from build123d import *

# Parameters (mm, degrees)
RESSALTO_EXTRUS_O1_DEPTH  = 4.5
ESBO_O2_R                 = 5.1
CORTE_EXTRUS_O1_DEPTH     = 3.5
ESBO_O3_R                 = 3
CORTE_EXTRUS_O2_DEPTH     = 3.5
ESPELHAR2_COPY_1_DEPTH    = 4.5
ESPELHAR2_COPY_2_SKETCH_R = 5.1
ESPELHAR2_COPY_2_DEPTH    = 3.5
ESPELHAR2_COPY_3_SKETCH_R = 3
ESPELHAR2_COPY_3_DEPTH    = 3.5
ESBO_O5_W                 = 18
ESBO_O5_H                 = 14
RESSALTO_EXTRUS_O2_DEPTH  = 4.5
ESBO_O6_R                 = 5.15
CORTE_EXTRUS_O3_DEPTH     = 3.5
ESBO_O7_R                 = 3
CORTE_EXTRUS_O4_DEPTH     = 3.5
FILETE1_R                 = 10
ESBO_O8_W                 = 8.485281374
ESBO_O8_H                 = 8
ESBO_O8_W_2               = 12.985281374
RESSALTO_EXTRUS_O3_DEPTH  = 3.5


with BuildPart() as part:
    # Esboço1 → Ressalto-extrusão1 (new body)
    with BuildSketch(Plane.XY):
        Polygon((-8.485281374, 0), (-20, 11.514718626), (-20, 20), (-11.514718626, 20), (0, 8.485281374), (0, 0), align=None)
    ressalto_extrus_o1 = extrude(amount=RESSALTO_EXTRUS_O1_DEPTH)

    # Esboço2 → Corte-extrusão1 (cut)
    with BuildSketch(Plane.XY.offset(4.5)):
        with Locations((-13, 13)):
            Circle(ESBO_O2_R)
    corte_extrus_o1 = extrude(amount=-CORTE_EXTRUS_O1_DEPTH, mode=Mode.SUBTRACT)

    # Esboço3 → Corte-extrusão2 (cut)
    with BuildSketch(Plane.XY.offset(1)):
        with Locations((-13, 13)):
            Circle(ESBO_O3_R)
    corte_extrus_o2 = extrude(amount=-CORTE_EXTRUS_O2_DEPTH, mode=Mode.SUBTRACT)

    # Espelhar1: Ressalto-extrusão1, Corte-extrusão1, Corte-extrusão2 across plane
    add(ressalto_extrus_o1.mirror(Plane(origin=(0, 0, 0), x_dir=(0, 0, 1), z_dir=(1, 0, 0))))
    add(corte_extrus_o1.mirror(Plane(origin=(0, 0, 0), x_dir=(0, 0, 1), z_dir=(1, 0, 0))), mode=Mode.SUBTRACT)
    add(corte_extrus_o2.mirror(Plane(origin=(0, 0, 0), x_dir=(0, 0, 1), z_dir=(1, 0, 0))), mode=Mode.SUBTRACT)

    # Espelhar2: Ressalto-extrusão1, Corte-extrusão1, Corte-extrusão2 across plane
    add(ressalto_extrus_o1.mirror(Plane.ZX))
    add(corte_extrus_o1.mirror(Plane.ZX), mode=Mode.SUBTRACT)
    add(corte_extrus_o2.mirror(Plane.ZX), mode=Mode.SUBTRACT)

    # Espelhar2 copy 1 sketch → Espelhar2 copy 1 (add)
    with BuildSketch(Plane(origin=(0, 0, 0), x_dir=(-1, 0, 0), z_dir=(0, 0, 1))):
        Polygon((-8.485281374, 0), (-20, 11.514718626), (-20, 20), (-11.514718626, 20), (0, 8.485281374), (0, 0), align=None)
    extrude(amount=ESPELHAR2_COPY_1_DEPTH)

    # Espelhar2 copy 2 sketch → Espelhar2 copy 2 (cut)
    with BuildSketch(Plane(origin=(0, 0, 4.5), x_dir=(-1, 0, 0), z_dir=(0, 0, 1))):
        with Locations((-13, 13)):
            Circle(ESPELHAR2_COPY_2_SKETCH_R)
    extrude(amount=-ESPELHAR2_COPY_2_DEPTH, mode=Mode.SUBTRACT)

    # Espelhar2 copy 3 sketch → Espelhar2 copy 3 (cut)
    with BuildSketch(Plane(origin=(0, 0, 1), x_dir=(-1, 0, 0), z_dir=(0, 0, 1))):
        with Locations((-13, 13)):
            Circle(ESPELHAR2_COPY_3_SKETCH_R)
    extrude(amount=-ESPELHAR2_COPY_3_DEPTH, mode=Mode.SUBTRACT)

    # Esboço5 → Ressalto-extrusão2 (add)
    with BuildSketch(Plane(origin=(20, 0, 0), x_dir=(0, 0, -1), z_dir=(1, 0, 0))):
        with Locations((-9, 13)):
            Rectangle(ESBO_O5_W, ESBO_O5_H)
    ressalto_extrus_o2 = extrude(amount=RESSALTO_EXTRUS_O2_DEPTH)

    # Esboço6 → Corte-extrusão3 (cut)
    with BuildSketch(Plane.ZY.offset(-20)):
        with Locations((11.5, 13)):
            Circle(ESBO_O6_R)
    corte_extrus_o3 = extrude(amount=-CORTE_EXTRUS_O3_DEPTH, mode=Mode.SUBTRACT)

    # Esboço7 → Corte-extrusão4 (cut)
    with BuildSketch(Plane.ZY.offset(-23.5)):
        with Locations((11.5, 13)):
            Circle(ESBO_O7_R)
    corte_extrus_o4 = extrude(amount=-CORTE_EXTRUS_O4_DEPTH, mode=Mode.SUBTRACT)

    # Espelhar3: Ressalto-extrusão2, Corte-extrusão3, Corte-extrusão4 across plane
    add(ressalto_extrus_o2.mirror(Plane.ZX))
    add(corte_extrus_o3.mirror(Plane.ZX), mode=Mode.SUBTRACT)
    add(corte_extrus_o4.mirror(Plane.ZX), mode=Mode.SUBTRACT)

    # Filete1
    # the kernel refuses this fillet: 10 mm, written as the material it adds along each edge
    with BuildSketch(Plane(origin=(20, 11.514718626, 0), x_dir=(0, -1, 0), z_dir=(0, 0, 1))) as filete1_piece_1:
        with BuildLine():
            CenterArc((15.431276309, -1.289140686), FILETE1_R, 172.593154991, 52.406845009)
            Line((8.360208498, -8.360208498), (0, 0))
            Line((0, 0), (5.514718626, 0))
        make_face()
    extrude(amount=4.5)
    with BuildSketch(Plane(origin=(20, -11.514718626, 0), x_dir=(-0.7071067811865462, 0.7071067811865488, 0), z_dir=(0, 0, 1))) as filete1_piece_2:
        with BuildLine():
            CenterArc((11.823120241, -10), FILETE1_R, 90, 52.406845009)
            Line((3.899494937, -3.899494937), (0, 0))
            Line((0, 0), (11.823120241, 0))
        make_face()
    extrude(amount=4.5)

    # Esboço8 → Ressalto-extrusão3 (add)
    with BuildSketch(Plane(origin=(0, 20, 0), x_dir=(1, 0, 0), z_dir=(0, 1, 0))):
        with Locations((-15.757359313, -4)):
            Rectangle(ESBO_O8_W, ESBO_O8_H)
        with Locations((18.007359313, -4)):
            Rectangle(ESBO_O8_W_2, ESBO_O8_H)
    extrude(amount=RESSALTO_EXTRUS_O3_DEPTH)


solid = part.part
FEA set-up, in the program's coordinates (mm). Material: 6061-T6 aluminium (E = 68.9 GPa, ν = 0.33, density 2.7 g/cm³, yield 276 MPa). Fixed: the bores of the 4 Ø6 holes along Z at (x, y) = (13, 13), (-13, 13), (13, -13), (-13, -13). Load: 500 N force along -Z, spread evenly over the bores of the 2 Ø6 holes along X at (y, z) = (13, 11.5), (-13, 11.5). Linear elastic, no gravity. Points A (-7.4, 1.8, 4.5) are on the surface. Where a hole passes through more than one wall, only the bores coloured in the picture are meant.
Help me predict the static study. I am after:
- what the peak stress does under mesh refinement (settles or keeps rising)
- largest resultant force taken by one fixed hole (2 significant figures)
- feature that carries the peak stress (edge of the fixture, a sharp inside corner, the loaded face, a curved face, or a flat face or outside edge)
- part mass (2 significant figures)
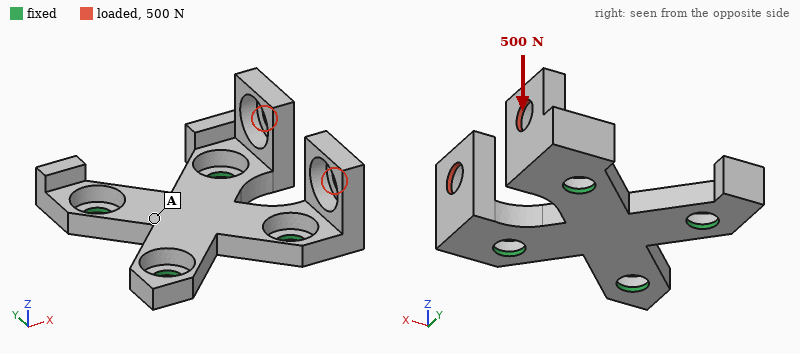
keeps rising
340 N
edge of the fixture
16 g
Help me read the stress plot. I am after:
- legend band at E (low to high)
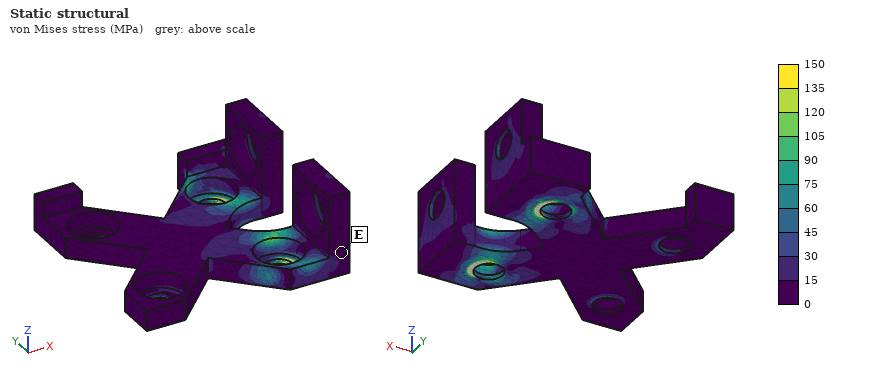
0 to 15 MPa
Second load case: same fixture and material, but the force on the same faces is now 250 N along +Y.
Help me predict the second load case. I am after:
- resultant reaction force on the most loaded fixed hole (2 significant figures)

130 N
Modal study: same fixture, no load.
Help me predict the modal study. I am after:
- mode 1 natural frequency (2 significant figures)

5400 Hz
